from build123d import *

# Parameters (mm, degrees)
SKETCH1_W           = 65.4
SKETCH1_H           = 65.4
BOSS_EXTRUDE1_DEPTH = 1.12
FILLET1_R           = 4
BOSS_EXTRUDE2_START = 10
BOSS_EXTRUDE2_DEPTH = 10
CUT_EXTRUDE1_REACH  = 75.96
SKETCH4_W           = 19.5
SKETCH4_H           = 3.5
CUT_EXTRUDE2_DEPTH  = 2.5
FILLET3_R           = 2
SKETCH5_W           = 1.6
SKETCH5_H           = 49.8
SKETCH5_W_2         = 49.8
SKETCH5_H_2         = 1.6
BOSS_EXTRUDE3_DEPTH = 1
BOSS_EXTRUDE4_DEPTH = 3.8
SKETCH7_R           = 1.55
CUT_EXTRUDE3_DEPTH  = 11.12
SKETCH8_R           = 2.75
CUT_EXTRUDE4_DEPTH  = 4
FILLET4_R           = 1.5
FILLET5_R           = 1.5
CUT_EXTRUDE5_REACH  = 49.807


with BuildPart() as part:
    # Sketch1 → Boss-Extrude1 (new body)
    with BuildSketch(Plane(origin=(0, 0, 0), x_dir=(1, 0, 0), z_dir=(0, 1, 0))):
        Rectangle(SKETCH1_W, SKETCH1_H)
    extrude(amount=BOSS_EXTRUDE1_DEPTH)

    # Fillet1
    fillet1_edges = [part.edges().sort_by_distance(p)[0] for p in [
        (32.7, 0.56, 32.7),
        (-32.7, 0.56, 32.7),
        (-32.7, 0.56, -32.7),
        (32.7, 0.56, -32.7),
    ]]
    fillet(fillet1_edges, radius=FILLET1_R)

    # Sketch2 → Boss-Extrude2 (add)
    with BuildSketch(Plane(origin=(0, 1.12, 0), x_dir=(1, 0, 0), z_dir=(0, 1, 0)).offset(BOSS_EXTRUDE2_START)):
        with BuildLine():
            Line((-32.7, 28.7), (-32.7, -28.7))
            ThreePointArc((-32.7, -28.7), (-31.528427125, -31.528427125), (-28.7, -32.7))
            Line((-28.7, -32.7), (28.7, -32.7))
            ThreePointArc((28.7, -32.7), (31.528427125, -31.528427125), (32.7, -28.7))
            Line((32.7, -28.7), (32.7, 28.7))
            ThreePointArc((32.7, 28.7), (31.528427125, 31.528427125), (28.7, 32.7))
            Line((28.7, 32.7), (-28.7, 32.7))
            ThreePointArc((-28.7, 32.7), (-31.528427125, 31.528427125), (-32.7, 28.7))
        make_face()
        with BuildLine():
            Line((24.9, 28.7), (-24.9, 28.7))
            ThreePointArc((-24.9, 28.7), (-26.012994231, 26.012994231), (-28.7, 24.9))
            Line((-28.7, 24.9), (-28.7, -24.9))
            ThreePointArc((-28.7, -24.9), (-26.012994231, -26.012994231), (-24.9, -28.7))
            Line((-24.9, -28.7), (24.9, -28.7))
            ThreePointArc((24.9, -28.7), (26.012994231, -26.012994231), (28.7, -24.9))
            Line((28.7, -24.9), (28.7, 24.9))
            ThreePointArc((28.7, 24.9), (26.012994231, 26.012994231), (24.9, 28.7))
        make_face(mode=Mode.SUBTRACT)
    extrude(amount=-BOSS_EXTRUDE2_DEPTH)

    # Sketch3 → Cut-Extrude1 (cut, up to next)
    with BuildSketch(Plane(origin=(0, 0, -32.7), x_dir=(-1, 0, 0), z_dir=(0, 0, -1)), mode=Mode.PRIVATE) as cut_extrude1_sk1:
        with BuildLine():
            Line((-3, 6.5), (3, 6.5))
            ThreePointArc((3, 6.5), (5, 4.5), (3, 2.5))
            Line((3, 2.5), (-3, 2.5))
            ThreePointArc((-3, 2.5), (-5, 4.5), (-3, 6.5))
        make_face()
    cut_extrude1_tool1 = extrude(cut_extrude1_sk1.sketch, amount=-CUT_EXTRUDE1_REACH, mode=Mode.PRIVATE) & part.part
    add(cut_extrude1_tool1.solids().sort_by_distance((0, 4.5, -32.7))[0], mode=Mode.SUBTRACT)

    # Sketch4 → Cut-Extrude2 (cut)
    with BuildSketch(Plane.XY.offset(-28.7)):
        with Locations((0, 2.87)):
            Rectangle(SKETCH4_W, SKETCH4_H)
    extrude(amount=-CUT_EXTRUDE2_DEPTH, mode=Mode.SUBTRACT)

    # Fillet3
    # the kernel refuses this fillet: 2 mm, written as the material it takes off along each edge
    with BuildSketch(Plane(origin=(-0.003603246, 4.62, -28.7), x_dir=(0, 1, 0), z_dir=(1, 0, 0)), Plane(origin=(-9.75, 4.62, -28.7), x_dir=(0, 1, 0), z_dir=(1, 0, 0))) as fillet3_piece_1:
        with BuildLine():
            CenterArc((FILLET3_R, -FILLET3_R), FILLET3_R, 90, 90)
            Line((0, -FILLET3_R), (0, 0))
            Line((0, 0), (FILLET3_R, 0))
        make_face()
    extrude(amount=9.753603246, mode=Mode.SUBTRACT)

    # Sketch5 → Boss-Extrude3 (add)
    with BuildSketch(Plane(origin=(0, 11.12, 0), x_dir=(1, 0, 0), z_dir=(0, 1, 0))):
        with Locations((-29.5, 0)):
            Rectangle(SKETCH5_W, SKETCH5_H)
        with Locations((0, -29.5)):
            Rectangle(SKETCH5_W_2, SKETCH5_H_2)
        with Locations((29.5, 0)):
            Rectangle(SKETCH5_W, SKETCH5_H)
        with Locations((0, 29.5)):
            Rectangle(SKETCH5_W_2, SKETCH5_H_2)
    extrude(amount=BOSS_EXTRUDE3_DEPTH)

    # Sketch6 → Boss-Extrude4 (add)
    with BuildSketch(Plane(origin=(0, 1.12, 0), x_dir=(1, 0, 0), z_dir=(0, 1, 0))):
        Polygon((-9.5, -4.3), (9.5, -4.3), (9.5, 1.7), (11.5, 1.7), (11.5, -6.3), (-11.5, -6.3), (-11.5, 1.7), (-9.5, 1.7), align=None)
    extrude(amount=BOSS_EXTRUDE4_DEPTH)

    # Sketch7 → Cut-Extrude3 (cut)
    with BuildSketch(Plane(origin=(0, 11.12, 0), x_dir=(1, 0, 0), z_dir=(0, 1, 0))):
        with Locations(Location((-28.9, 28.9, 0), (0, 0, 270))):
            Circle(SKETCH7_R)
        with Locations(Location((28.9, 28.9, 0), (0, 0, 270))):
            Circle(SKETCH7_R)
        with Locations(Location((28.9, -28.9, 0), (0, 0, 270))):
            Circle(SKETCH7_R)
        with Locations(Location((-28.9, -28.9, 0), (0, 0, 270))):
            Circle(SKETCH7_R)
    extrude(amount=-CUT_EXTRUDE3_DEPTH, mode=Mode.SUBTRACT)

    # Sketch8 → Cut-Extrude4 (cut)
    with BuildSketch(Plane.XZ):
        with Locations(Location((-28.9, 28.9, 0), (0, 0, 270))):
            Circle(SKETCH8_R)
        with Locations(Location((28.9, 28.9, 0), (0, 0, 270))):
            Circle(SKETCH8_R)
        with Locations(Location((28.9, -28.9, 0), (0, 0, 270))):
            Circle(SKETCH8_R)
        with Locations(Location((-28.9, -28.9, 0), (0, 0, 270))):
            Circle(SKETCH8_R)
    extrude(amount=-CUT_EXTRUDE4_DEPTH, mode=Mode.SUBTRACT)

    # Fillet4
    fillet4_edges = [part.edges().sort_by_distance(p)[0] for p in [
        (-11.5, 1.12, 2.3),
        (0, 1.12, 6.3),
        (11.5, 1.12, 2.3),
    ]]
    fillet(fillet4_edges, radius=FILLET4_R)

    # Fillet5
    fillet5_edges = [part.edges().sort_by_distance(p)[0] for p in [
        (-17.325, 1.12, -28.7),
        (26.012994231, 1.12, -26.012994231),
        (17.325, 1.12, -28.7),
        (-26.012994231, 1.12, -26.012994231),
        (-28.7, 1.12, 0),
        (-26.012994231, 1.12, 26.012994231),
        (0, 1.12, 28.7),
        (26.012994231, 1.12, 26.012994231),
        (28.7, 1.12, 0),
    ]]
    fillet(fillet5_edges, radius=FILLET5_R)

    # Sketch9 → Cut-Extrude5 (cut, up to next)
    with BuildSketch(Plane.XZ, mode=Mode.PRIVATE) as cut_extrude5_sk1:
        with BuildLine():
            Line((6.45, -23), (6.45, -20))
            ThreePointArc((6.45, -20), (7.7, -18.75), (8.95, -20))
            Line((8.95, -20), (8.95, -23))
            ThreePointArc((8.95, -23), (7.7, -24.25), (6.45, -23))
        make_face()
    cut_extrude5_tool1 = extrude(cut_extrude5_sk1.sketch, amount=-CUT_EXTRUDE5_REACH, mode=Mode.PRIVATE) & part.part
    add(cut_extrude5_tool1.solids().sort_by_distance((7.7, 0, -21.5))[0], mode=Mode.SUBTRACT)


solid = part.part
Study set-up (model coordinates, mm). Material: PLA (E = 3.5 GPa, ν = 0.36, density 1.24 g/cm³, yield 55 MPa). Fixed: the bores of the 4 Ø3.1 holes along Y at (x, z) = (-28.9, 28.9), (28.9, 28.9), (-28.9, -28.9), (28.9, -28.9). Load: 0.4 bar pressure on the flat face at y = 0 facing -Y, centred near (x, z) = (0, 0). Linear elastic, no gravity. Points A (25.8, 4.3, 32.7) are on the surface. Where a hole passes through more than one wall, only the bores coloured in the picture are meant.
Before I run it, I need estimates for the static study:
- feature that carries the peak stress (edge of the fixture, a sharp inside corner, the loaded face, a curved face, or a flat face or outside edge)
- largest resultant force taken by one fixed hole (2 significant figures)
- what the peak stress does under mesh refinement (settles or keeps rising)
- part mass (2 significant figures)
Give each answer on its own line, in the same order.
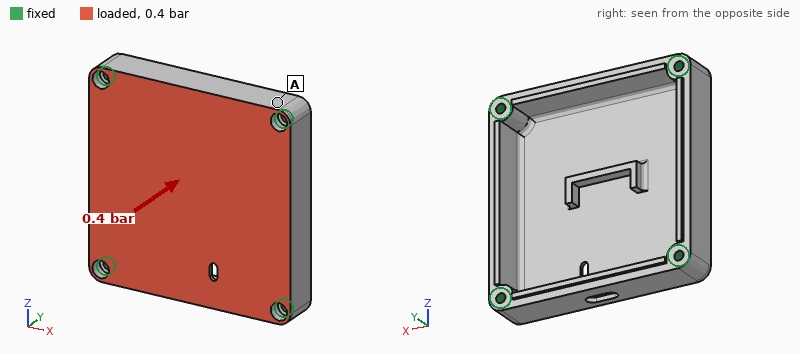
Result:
a sharp inside corner
53 N
keeps rising
18 g
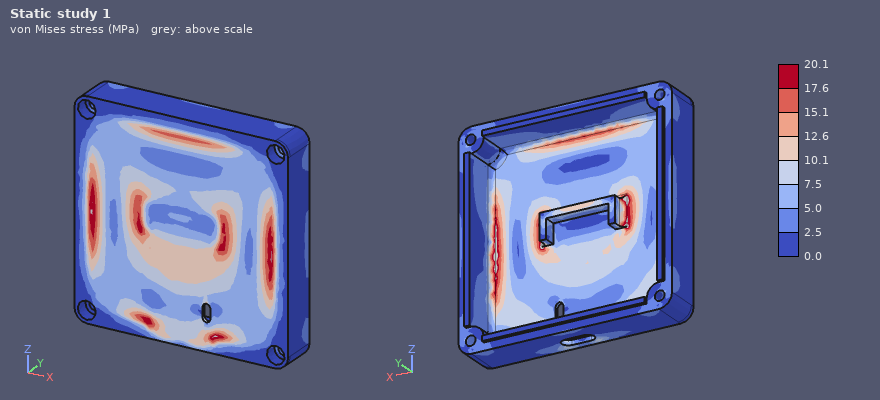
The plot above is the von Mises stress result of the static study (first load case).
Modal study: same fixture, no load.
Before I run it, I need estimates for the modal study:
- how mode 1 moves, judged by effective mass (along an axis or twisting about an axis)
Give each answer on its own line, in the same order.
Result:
along Y
